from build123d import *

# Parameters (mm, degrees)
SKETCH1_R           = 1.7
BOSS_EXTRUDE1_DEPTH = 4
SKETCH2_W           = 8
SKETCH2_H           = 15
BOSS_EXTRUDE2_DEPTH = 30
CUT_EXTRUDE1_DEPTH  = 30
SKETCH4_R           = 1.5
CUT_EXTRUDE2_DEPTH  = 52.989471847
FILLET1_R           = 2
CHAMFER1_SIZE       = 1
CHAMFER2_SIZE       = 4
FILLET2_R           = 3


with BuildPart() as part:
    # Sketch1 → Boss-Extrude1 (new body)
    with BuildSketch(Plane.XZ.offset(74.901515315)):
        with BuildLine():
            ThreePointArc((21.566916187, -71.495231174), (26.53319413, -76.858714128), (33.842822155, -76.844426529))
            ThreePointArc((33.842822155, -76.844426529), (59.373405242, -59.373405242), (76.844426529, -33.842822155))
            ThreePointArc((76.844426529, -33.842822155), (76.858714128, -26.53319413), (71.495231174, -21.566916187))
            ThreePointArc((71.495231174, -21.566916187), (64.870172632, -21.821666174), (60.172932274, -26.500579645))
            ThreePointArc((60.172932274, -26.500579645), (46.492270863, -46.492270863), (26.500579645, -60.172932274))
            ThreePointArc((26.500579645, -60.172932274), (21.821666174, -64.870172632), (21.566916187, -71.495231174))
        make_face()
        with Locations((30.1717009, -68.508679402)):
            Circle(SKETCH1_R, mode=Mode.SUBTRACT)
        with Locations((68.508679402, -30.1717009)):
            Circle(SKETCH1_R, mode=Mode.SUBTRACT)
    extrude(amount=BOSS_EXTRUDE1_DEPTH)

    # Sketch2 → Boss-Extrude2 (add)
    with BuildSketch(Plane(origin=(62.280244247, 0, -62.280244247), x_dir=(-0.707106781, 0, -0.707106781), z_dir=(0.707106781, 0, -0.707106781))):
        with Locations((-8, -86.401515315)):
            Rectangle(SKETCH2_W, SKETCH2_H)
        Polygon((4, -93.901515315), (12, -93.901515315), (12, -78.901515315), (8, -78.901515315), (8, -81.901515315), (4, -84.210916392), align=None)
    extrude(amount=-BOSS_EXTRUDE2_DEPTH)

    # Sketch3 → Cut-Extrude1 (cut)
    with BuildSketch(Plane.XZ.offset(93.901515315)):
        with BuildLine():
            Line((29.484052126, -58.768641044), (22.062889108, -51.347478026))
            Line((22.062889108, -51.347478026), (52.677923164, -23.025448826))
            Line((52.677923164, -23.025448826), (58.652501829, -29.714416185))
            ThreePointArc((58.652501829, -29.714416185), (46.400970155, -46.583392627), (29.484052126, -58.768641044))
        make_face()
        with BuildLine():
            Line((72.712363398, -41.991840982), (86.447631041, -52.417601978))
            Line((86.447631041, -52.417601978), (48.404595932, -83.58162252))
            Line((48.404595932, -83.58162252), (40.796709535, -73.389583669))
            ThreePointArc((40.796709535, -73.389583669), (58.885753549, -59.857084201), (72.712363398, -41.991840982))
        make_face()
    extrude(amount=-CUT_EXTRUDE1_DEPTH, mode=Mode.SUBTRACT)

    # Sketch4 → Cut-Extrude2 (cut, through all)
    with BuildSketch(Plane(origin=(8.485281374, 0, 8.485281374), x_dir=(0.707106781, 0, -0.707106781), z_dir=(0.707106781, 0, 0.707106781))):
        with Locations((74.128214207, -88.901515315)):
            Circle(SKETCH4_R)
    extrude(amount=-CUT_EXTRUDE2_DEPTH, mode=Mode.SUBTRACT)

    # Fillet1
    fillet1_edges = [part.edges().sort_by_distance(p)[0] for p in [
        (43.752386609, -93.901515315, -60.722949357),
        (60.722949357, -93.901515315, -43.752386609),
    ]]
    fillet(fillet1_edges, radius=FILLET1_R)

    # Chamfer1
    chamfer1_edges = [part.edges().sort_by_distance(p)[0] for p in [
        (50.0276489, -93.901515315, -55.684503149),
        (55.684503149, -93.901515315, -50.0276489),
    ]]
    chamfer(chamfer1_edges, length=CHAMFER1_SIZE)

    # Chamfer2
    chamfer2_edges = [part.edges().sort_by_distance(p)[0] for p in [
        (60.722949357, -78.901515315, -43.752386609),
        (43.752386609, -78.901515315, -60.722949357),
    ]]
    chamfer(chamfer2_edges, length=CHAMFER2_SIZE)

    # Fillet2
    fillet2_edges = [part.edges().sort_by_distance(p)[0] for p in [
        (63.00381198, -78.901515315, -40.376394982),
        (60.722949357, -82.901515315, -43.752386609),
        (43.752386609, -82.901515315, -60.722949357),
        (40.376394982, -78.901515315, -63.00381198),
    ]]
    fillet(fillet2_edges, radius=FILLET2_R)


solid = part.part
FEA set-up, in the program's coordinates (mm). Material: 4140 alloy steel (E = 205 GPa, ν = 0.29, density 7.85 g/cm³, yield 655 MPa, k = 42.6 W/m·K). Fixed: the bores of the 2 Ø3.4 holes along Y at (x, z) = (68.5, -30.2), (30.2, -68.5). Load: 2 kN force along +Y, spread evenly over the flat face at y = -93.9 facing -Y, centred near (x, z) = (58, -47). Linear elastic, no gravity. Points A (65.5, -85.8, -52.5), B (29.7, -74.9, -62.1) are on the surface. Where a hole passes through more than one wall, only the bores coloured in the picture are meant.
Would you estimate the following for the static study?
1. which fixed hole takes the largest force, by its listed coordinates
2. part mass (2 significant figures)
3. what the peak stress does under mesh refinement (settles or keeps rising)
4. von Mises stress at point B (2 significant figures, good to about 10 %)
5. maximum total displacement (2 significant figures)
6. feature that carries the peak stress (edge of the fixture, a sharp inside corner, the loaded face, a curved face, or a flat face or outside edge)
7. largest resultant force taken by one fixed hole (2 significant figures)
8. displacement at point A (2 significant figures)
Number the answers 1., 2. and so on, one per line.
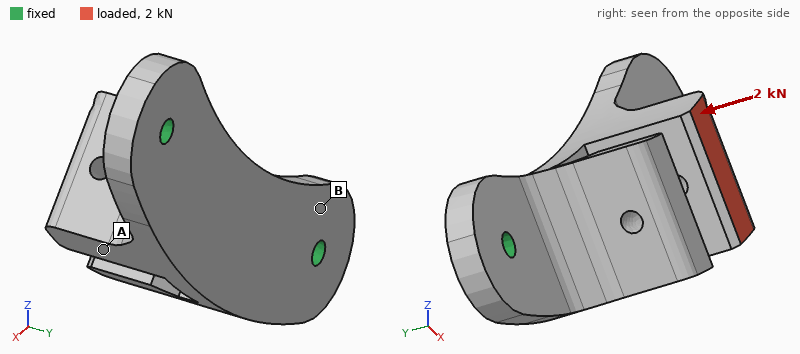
1. (68.5, -30.2)
2. 73 g
3. keeps rising
4. 110 MPa
5. 0.10 mm
6. edge of the fixture
7. 1.4 kN
8. 0.080 mm
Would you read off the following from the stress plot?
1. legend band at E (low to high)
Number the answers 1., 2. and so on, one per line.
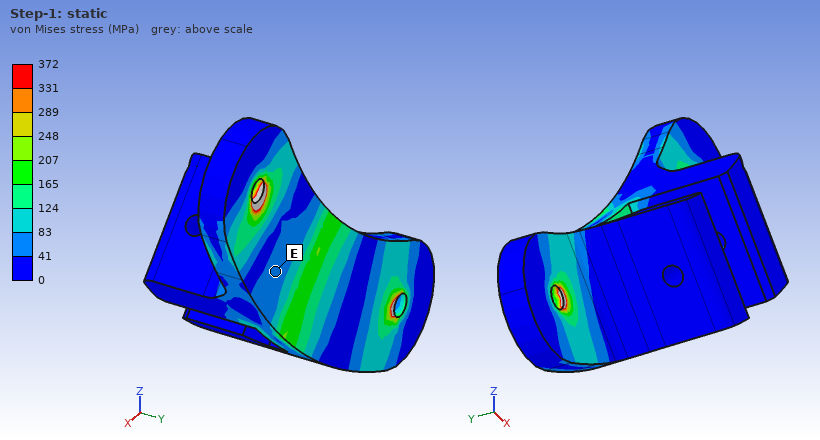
1. 41 to 83 MPa
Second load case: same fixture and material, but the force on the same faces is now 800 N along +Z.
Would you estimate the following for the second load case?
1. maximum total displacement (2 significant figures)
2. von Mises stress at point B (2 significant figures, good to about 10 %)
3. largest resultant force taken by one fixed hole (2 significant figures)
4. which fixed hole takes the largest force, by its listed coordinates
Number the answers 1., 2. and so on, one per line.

1. 74 µm
2. 42 MPa
3. 790 N
4. (68.5, -30.2)
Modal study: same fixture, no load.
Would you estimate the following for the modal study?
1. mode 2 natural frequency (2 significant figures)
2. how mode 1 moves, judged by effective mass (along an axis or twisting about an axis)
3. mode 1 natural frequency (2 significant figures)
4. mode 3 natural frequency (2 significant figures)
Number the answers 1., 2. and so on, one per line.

1. 4900 Hz
2. along Y
3. 3500 Hz
4. 8500 Hz
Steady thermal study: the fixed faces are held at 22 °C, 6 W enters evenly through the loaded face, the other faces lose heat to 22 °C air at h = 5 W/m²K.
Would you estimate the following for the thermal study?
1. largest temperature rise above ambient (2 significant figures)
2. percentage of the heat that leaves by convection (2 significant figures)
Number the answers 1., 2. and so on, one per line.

1. 36 K
2. 5.0 %
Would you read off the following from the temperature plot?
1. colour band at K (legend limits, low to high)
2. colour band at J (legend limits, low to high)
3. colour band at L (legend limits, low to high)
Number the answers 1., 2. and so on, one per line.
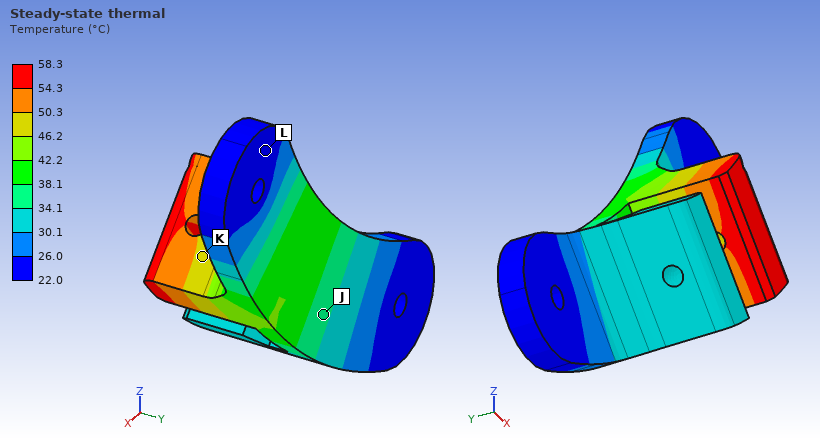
1. 46.2 to 50.3 °C
2. 34.1 to 38.1 °C
3. 22.0 to 26.0 °C
